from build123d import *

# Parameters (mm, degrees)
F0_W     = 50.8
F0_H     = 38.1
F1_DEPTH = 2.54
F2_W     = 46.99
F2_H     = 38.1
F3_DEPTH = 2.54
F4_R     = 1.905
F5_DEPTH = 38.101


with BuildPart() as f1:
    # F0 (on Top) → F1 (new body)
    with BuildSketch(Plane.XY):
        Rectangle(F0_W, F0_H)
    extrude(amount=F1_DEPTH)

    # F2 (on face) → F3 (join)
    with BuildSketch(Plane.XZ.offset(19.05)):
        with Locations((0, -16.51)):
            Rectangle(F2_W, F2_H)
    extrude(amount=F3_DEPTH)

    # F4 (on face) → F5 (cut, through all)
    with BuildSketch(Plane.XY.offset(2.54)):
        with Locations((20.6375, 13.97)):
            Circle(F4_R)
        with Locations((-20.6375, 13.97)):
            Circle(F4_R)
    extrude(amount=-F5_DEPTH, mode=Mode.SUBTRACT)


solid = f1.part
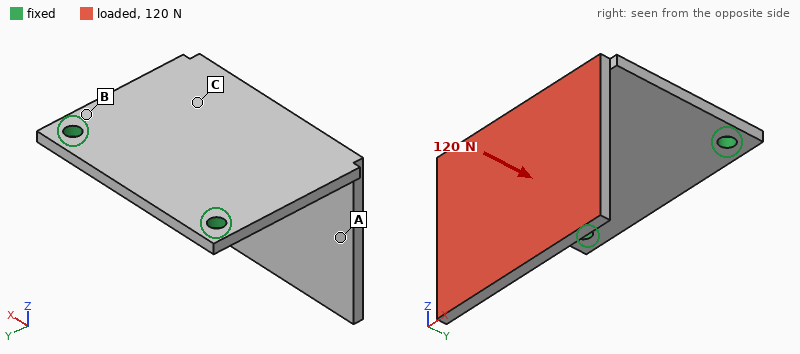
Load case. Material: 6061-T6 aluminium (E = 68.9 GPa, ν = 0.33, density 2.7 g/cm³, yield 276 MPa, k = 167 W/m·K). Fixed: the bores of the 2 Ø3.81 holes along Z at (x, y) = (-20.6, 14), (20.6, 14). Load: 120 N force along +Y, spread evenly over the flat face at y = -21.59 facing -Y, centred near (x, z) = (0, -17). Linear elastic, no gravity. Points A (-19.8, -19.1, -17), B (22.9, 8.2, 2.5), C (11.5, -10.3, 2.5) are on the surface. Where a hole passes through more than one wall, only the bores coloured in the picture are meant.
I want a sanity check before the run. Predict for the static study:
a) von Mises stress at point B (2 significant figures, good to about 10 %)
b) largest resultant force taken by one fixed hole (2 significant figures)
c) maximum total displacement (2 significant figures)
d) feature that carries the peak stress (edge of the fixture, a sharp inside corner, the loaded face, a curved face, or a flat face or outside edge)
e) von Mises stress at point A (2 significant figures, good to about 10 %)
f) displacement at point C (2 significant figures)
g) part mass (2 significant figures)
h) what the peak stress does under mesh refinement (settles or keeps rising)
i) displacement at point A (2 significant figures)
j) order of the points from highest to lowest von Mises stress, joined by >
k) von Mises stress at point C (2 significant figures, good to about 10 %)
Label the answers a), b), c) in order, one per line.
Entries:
a) 54 MPa
b) 63 N
c) 0.79 mm
d) edge of the fixture
e) 10 MPa
f) 0.16 mm
g) 25 g
h) keeps rising
i) 0.43 mm
j) B > C > A
k) 34 MPa
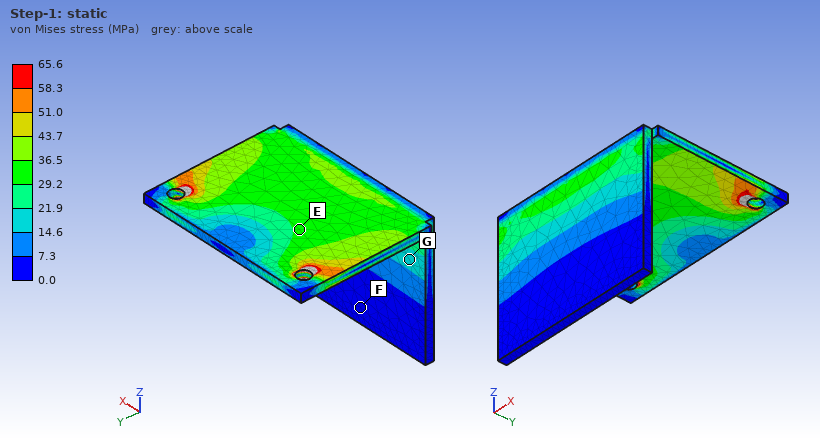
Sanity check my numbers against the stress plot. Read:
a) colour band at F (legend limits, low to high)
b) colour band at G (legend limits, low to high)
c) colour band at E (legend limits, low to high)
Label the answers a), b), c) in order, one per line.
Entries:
a) 0.0 to 7.3 MPa
b) 14.6 to 21.9 MPa
c) 29.2 to 36.5 MPa
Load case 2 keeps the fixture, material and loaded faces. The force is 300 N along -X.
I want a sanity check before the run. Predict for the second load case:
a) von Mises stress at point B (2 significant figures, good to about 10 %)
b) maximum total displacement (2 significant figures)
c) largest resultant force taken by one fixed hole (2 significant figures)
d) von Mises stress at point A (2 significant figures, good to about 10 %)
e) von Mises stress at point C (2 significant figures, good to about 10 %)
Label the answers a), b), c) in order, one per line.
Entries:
a) 84 MPa
b) 0.57 mm
c) 320 N
d) 13 MPa
e) 50 MPa
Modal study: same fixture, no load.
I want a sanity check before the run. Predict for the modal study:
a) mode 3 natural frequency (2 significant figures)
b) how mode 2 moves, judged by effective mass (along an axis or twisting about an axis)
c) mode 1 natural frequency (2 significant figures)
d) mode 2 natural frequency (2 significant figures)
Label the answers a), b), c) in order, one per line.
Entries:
a) 1500 Hz
b) along X
c) 540 Hz
d) 1100 Hz
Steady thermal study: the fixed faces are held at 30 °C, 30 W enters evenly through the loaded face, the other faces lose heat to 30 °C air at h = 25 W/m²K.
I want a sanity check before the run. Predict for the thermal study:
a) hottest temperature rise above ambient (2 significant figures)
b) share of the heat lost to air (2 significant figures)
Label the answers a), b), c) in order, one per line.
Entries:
a) 70 K
b) 19 %
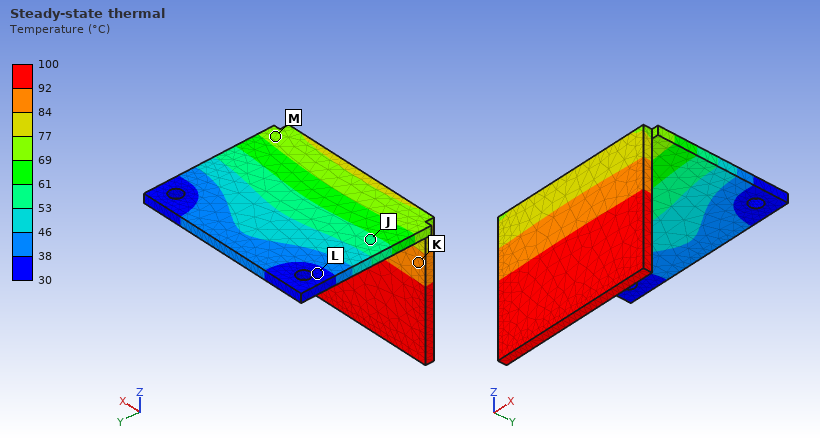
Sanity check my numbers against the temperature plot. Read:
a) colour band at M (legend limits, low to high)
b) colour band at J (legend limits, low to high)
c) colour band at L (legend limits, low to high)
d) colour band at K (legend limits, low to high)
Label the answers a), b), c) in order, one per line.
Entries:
a) 69 to 77 °C
b) 53 to 61 °C
c) 30 to 38 °C
d) 84 to 92 °C
